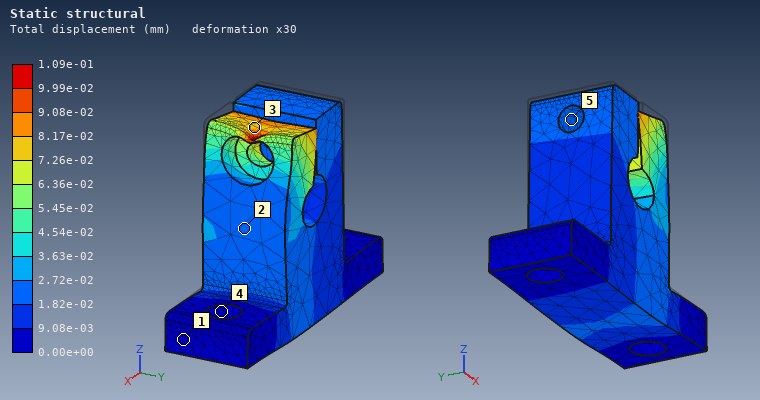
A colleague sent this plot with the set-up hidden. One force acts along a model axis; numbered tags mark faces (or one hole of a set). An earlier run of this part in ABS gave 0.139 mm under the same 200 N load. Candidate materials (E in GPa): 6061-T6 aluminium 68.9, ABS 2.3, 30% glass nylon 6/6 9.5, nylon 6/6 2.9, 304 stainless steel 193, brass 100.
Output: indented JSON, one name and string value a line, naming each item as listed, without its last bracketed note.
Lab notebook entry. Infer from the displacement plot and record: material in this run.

{
  "material in this run": "nylon 6/6"
}
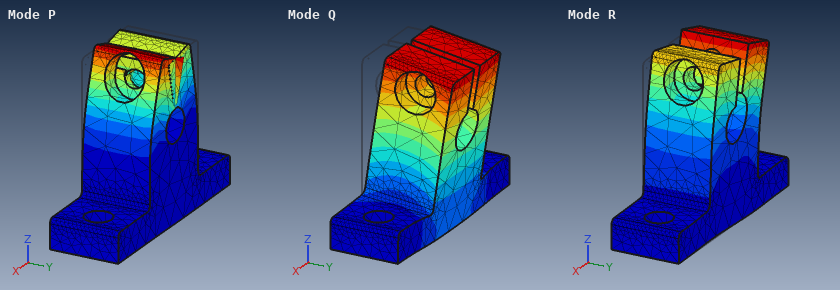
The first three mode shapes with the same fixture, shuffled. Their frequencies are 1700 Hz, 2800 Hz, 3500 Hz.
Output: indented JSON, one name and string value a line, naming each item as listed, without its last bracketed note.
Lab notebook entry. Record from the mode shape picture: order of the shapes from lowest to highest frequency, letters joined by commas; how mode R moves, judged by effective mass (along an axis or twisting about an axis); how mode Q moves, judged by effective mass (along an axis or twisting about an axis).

{
  "order of the shapes from lowest to highest frequency, letters joined by commas": "Q, R, P",
  "how mode R moves, judged by effective mass": "along X",
  "how mode Q moves, judged by effective mass": "along Y"
}
